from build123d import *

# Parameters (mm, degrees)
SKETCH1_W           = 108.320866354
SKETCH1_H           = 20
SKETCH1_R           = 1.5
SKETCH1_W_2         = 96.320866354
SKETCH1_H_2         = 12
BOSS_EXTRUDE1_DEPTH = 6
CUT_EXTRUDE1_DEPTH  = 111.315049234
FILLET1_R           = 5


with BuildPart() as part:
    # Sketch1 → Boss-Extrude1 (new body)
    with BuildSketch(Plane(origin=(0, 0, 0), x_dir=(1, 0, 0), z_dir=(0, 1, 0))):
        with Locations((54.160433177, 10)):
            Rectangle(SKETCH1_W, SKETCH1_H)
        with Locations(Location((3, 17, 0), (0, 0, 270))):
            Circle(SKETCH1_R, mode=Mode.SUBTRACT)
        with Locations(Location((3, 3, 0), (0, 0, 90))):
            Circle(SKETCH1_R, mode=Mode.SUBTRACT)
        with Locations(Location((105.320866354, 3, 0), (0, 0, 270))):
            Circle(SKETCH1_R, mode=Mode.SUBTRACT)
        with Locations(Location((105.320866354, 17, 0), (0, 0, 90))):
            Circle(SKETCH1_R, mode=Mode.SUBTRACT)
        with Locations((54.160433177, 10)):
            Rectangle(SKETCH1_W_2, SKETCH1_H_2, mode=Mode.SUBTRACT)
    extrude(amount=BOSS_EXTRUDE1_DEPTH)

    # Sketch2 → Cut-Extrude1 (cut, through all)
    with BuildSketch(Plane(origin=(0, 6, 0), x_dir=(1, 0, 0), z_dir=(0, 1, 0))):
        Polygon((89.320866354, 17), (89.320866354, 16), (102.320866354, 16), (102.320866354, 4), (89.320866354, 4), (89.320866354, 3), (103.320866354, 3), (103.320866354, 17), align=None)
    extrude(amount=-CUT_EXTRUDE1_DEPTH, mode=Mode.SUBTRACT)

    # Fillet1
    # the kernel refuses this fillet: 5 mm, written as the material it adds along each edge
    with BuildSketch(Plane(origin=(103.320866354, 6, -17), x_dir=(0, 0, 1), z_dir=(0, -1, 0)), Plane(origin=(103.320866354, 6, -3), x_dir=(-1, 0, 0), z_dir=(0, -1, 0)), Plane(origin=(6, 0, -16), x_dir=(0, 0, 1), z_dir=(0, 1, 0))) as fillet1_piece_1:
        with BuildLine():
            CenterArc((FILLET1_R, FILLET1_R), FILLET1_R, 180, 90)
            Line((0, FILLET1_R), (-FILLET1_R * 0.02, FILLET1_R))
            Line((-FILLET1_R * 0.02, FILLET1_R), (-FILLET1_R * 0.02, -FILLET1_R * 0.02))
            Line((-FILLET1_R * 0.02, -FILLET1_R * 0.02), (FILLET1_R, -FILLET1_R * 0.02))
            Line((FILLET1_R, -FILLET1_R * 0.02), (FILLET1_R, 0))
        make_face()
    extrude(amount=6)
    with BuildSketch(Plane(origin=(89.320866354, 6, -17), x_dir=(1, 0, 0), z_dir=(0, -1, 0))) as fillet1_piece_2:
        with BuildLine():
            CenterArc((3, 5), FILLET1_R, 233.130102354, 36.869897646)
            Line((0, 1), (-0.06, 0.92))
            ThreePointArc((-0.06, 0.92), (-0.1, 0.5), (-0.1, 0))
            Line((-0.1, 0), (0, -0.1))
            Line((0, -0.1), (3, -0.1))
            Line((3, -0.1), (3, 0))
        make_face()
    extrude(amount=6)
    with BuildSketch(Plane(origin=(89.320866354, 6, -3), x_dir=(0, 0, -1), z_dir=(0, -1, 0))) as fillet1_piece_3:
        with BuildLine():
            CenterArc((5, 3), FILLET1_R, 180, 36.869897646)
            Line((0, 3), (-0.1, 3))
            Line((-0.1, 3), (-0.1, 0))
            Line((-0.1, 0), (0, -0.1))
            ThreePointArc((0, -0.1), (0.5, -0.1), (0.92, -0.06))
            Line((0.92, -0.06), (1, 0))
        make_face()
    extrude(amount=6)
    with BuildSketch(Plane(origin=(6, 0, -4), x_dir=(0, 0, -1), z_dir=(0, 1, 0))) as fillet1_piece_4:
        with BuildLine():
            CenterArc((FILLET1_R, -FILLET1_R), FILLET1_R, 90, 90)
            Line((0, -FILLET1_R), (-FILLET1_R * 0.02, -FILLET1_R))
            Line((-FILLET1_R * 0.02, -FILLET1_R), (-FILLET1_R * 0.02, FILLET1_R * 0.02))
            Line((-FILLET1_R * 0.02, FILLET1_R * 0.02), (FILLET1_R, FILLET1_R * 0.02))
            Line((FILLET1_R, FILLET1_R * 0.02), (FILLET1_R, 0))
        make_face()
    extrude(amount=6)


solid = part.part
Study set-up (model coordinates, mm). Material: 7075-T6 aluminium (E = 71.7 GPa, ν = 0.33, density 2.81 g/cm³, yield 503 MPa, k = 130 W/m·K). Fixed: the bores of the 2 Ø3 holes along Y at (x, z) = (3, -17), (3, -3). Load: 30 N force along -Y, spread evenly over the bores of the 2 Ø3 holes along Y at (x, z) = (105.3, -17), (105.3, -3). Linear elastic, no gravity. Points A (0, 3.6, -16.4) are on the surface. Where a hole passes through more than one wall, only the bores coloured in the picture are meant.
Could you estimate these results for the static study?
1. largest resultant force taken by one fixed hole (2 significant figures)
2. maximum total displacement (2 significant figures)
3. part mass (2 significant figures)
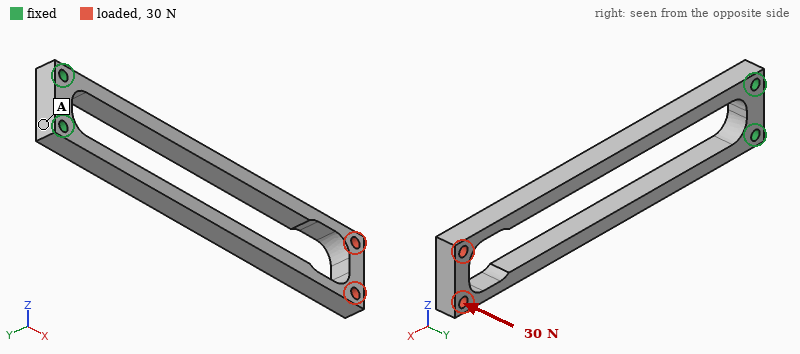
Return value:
15 N
1.0 mm
16 g
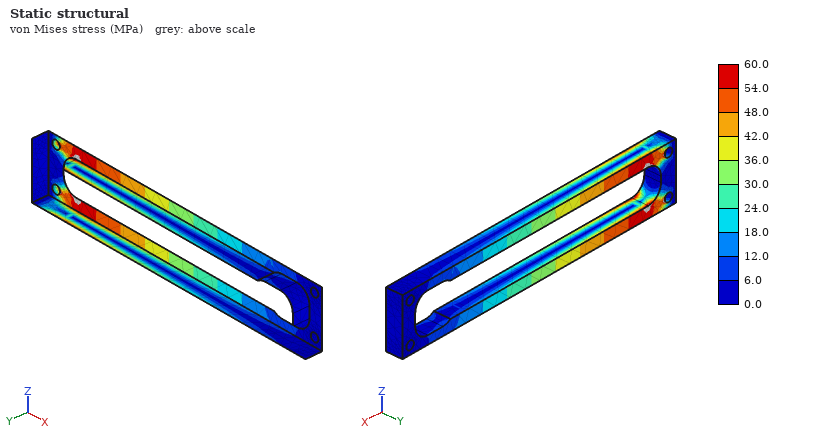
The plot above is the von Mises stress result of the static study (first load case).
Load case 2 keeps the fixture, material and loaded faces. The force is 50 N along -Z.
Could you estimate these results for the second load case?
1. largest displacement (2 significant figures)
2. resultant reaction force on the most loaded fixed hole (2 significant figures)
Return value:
1.2 mm
250 N
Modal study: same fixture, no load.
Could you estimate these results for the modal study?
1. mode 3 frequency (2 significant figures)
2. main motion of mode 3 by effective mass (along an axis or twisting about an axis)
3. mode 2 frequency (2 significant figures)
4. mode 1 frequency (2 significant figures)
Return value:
1700 Hz
twisting about X
440 Hz
420 Hz
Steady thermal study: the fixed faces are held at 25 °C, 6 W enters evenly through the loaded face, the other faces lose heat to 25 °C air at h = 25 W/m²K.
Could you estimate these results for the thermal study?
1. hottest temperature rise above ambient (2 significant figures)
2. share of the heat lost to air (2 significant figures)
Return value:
62 K
52 %
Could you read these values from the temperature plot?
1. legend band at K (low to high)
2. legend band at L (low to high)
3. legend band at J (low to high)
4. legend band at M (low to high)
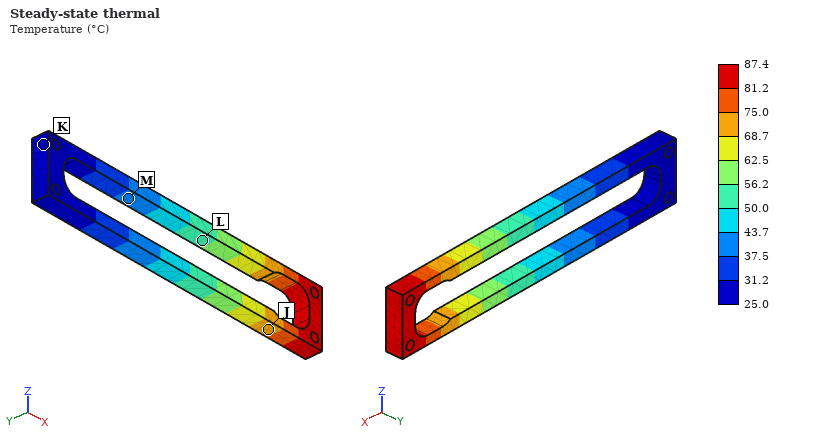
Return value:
25.0 to 31.2 °C
50.0 to 56.2 °C
68.7 to 75.0 °C
37.5 to 43.7 °C
